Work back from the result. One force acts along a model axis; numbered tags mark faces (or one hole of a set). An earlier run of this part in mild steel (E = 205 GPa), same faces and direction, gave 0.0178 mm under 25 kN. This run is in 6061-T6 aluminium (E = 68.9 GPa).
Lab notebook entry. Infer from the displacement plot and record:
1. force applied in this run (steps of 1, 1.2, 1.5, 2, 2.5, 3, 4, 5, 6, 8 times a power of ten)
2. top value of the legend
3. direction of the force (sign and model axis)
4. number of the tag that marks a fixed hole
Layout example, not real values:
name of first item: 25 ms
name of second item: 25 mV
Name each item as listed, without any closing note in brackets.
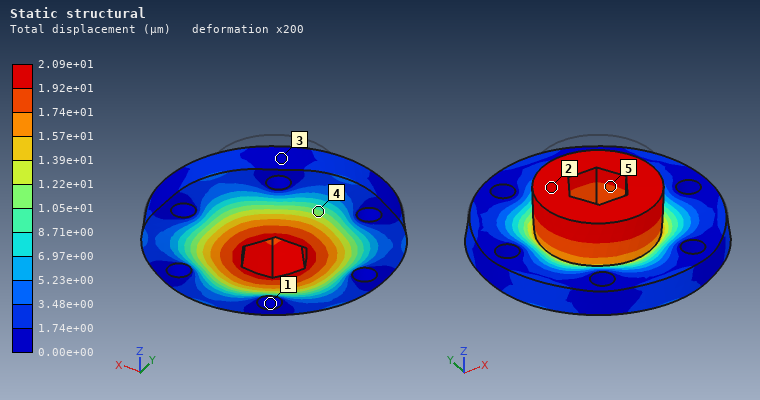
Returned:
force applied in this run: 10 kN
top value of the legend: 2.09e+01 µm
direction of the force: -Z
number of the tag that marks a fixed hole: 1
